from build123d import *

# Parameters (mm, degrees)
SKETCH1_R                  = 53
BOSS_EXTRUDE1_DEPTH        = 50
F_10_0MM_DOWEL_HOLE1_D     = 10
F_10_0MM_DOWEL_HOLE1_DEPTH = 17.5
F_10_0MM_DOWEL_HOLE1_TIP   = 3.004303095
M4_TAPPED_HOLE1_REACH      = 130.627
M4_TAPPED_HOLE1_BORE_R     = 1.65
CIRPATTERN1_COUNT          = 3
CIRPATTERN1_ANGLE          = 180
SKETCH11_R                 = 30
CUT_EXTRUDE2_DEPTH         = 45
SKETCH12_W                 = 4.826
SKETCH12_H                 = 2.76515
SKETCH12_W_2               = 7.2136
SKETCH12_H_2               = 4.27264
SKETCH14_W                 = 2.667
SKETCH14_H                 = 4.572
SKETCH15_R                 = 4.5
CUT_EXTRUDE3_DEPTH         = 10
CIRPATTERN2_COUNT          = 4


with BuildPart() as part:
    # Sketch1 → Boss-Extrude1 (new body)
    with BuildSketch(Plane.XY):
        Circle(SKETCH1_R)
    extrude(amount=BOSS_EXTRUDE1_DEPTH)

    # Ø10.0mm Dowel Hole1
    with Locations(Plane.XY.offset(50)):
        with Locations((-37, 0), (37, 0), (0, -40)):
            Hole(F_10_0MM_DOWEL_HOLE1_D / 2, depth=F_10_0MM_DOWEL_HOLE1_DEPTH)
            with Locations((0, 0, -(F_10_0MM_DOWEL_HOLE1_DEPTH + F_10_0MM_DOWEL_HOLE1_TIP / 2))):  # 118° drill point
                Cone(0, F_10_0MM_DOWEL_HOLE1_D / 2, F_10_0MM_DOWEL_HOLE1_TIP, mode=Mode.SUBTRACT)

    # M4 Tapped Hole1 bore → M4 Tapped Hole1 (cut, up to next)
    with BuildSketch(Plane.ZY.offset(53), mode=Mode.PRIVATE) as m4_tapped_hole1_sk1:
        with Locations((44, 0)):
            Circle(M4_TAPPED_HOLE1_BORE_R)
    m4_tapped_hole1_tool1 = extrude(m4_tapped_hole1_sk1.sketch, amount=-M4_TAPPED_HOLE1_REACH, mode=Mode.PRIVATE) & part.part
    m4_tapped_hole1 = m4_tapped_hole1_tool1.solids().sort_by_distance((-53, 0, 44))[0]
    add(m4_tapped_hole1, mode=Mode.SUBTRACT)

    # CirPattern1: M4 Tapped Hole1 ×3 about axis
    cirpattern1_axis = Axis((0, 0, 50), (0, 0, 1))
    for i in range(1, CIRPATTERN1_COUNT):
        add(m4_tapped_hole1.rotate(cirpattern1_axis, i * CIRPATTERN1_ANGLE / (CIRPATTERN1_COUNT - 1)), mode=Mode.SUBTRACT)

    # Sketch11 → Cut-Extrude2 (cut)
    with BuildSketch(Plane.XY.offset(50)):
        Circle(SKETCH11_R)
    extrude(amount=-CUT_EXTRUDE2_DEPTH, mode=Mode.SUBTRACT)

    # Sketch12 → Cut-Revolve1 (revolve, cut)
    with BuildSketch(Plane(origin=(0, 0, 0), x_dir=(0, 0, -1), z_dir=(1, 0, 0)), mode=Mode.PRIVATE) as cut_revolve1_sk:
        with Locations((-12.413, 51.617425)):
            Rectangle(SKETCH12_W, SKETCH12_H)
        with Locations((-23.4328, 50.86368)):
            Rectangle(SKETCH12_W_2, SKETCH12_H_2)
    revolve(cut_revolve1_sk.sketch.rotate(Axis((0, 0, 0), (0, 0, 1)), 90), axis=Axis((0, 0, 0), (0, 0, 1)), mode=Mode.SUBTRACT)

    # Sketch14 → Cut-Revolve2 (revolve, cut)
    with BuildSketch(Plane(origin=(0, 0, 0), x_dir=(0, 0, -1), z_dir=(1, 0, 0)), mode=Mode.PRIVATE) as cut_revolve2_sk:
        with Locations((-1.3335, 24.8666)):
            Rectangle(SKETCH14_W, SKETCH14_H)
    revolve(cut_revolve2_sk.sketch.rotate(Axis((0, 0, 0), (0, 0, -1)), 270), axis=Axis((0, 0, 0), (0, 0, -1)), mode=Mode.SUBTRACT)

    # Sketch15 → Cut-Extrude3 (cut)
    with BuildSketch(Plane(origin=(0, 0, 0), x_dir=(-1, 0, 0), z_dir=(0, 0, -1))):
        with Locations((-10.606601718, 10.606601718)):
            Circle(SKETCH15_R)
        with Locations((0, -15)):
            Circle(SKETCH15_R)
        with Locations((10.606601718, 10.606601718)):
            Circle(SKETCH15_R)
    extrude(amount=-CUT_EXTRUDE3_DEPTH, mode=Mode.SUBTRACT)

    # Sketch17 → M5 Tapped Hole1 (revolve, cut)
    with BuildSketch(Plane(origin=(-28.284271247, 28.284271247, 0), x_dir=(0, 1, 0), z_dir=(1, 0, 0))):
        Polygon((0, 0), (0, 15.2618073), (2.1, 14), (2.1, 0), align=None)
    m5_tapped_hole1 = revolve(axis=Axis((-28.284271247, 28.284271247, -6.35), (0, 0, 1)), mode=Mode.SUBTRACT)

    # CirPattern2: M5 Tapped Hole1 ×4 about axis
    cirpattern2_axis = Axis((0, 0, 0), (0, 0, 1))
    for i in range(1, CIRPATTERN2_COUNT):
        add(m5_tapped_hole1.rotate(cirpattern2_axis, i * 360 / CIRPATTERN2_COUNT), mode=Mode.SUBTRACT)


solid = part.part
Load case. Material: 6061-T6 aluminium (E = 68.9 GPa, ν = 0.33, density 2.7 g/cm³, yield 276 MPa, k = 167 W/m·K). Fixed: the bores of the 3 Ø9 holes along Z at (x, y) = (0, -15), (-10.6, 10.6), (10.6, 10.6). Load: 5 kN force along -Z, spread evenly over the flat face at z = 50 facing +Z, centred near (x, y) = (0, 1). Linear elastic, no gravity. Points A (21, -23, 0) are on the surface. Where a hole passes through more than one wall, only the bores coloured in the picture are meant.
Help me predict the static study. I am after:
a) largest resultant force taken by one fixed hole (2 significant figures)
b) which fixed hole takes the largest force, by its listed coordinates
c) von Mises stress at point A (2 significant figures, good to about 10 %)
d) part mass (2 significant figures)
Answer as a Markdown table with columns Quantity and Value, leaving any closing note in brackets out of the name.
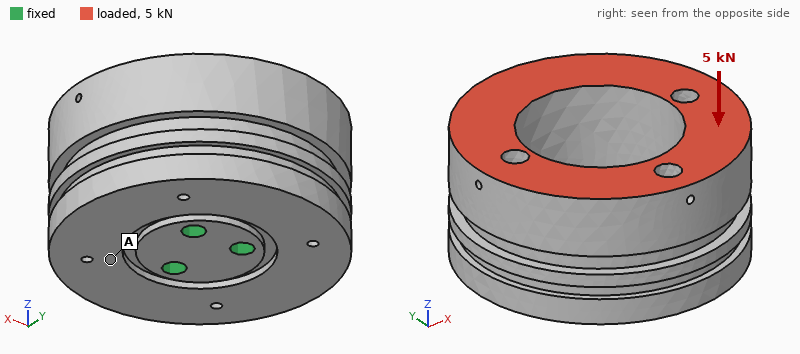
| Quantity | Value |
|---|---|
| largest resultant force taken by one fixed hole | 2.0 kN |
| which fixed hole takes the largest force, by its listed coordinates | (0, -15) |
| von Mises stress at point A | 16 MPa |
| part mass | 790 g |
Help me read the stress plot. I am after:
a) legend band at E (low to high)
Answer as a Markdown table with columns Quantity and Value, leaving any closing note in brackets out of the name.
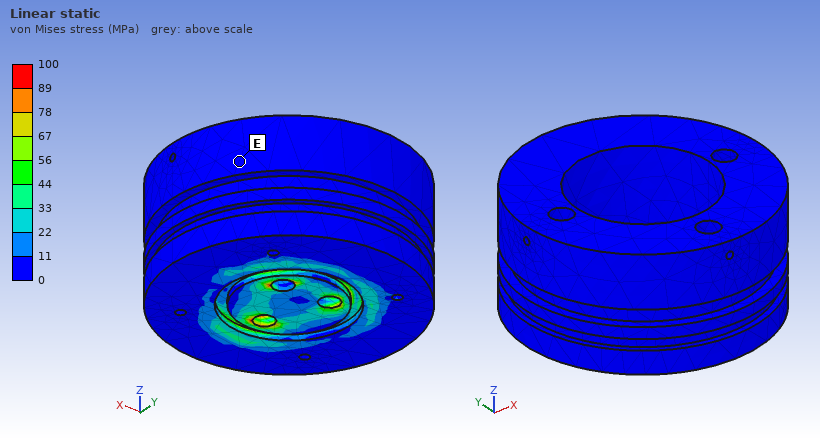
| Quantity | Value |
|---|---|
| legend band at E | 0 to 11 MPa |
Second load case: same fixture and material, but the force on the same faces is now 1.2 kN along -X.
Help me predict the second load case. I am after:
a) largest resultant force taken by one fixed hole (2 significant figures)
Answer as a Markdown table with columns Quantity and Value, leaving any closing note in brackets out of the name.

| Quantity | Value |
|---|---|
| largest resultant force taken by one fixed hole | 1.4 kN |
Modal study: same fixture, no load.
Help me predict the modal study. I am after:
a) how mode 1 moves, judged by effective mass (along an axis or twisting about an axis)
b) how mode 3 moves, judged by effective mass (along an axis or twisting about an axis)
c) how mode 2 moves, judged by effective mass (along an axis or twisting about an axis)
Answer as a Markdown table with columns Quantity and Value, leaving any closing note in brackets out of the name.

| Quantity | Value |
|---|---|
| how mode 1 moves, judged by effective mass | along X |
| how mode 3 moves, judged by effective mass | along Z |
| how mode 2 moves, judged by effective mass | along Y |
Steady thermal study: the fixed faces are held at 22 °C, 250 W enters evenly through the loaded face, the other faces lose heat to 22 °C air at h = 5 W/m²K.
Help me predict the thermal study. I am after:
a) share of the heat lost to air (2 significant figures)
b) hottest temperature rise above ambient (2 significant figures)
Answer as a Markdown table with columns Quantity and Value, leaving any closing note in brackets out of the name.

| Quantity | Value |
|---|---|
| share of the heat lost to air | 4.8 % |
| hottest temperature rise above ambient | 66 K |
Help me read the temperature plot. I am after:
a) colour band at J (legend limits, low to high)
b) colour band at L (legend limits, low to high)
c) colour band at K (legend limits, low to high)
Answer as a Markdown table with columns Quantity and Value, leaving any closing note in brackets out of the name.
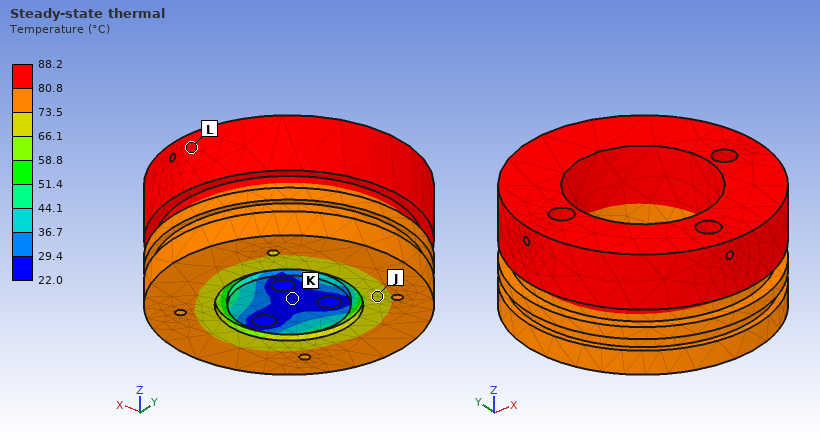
| Quantity | Value |
|---|---|
| colour band at J | 66.1 to 73.5 °C |
| colour band at L | 80.8 to 88.2 °C |
| colour band at K | 22.0 to 29.4 °C |
